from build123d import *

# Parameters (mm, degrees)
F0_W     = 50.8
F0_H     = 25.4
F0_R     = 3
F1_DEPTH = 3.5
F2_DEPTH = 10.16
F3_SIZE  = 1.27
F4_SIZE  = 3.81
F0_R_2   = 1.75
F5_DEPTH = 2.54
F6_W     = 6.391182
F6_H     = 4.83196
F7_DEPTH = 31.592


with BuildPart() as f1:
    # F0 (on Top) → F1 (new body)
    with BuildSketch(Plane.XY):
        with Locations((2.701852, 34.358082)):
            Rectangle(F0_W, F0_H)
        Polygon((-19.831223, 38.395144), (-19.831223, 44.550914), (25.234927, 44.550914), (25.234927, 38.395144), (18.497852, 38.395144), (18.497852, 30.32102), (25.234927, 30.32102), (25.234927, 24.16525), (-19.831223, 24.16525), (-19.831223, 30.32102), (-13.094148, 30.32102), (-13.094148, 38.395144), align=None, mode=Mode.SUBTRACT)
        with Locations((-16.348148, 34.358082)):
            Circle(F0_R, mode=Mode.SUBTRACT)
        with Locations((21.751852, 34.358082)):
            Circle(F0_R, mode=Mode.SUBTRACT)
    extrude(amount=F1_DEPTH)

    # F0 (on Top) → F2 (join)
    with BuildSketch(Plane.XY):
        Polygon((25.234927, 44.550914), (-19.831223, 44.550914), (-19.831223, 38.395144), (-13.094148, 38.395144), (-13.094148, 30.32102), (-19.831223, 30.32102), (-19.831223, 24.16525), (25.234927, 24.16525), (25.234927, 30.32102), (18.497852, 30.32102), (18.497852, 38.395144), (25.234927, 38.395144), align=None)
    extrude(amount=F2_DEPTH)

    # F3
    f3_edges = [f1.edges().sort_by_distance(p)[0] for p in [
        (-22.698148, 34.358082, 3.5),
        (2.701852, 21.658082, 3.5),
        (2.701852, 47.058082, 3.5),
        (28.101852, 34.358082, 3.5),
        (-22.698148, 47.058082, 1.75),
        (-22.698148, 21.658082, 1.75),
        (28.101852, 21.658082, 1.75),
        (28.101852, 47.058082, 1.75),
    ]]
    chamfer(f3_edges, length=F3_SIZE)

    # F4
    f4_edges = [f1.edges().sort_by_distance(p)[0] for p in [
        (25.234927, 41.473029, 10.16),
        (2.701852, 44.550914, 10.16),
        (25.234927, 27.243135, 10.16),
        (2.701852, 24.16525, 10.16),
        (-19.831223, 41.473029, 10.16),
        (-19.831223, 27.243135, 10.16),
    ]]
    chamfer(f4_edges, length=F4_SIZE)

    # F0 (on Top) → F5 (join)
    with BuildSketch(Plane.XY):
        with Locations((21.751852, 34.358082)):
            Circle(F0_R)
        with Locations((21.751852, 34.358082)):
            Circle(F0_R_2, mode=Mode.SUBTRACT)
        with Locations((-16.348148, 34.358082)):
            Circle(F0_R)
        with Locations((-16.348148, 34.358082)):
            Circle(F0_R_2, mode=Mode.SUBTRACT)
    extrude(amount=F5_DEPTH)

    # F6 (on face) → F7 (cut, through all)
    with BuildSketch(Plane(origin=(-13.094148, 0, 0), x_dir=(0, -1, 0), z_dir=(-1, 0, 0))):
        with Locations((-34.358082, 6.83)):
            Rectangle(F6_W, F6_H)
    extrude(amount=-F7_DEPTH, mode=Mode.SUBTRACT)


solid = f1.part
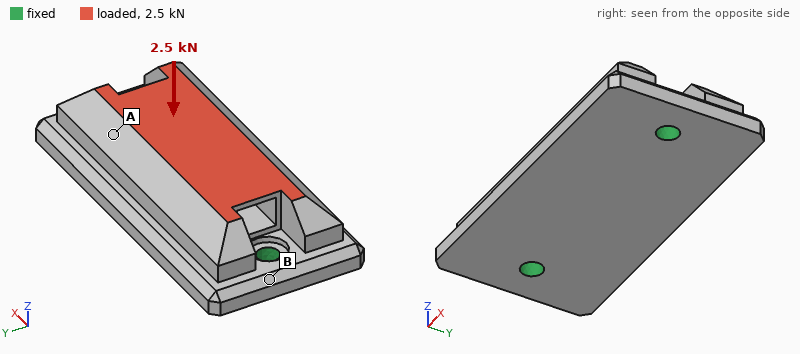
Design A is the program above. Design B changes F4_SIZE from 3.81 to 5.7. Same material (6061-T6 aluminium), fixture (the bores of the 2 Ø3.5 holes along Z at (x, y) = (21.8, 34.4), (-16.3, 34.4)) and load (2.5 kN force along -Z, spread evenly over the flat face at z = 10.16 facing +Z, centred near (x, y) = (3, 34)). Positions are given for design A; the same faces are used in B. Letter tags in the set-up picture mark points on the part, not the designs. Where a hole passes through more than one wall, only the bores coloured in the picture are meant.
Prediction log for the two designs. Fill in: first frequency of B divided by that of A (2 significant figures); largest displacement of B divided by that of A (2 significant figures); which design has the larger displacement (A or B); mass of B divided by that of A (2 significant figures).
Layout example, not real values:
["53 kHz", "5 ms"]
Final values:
["1.1", "1.3", "B", "0.89"]
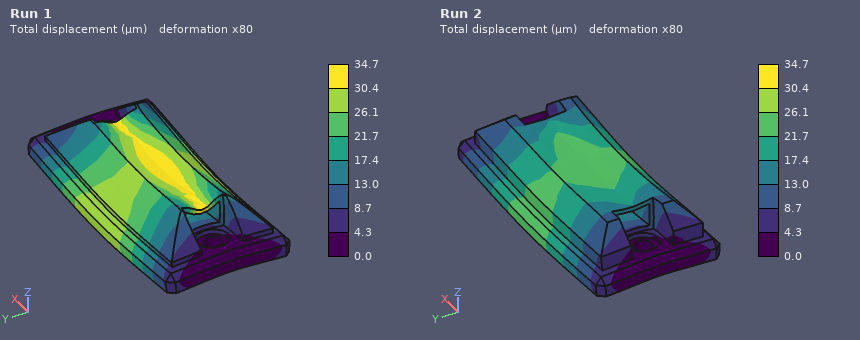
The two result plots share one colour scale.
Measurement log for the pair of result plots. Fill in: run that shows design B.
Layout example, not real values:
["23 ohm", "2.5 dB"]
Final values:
["Run 1"]
